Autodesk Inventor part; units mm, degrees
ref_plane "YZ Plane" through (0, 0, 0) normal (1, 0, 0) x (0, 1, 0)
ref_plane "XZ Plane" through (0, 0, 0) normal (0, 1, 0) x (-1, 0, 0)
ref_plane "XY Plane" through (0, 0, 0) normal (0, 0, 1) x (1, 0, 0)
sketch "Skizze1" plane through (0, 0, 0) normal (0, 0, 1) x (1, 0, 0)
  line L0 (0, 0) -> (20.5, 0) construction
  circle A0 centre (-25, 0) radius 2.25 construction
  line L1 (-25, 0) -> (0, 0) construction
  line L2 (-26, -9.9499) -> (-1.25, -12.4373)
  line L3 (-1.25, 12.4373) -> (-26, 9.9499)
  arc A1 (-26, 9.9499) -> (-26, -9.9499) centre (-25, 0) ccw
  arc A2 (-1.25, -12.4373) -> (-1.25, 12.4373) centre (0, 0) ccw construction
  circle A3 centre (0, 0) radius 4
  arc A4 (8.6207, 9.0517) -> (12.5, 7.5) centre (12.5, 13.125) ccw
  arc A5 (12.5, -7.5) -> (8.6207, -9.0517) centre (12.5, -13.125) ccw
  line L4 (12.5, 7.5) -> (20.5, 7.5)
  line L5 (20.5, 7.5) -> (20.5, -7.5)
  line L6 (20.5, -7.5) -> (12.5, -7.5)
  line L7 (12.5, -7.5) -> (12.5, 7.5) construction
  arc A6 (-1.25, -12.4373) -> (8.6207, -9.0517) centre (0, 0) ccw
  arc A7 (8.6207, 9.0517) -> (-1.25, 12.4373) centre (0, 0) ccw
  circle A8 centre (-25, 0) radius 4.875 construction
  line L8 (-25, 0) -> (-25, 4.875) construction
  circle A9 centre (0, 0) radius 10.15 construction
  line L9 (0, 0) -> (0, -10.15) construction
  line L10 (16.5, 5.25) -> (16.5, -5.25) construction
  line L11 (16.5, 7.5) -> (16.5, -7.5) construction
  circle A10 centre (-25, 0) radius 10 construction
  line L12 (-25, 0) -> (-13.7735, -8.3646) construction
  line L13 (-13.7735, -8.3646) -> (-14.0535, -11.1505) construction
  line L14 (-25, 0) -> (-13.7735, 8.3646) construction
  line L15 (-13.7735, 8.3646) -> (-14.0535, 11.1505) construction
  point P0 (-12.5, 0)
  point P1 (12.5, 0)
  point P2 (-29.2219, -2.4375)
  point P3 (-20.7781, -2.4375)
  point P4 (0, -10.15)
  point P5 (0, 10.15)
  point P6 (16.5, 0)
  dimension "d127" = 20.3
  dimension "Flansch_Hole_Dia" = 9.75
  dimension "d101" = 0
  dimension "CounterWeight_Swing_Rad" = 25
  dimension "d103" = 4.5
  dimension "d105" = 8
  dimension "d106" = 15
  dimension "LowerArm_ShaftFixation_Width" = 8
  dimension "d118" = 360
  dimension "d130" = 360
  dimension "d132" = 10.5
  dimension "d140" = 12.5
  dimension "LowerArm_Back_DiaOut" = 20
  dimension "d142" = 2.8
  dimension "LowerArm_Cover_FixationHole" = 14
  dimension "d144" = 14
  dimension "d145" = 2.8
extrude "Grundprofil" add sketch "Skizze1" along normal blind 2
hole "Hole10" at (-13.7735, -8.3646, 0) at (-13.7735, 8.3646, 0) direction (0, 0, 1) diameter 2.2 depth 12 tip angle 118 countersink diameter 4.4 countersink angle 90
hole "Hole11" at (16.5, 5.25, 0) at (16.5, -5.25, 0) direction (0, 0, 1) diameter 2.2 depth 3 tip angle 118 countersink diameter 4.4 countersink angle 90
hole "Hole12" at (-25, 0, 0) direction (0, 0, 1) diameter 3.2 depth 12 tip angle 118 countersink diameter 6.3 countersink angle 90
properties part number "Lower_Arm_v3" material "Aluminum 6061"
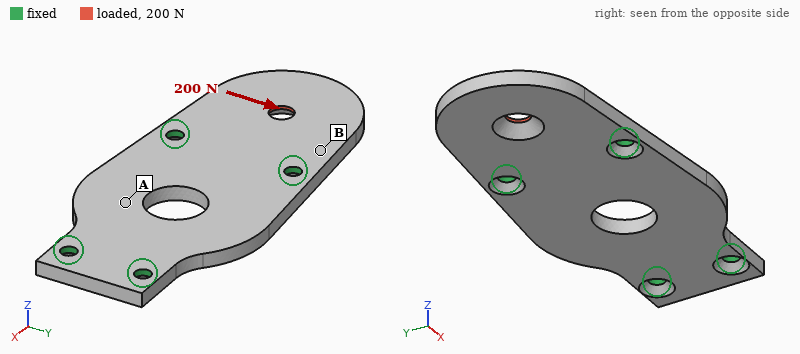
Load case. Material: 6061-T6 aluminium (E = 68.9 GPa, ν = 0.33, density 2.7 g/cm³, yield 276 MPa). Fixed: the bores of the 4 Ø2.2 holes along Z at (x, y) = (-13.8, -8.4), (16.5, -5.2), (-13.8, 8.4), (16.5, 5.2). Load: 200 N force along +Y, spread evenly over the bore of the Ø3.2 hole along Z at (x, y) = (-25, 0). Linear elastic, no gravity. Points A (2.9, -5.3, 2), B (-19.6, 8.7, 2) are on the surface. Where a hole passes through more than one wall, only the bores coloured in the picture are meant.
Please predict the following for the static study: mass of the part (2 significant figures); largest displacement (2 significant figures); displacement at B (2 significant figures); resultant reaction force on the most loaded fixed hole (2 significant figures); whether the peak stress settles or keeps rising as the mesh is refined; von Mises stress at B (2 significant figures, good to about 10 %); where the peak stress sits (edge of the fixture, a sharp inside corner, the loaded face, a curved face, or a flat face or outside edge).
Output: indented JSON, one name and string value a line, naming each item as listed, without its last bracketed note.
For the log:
{
  "mass of the part": "5.4 g",
  "largest displacement": "11 µm",
  "displacement at B": "4.2 µm",
  "resultant reaction force on the most loaded fixed hole": "150 N",
  "whether the peak stress settles or keeps rising as the mesh is refined": "keeps rising",
  "von Mises stress at B": "13 MPa",
  "where the peak stress sits": "edge of the fixture"
}
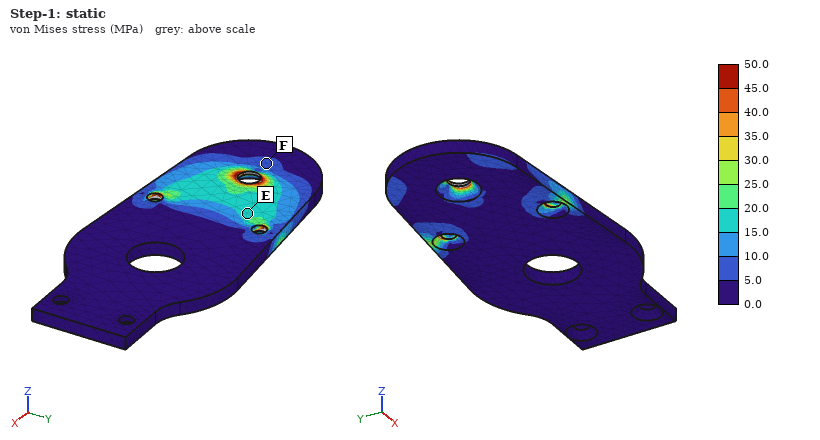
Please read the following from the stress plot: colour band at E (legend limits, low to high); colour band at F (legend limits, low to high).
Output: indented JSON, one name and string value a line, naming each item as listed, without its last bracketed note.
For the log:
{
  "colour band at E": "15.0 to 20.0 MPa",
  "colour band at F": "5.0 to 10.0 MPa"
}
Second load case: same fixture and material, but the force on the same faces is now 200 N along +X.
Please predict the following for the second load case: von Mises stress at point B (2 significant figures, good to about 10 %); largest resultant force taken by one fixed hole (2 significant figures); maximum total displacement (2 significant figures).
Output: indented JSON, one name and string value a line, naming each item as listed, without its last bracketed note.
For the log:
{
  "von Mises stress at point B": "15 MPa",
  "largest resultant force taken by one fixed hole": "96 N",
  "maximum total displacement": "30 µm"
}
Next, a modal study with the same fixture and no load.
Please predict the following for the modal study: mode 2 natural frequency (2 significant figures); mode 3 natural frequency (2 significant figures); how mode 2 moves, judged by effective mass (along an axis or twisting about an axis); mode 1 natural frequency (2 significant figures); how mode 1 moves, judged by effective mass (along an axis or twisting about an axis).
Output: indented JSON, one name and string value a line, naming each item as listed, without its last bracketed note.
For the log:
{
  "mode 2 natural frequency": "8900 Hz",
  "mode 3 natural frequency": "11 kHz",
  "how mode 2 moves, judged by effective mass": "along Z",
  "mode 1 natural frequency": "3600 Hz",
  "how mode 1 moves, judged by effective mass": "along Z"
}
